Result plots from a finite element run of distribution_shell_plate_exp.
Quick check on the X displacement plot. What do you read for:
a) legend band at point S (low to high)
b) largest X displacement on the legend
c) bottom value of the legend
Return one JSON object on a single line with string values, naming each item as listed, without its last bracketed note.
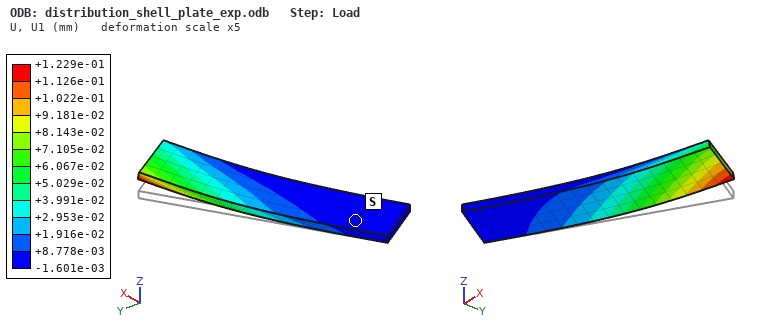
{"legend band at point S": "-1.601e-03 to +8.778e-03 mm", "largest X displacement on the legend": "+1.229e-01 mm", "bottom value of the legend": "-1.601e-03 mm"}
